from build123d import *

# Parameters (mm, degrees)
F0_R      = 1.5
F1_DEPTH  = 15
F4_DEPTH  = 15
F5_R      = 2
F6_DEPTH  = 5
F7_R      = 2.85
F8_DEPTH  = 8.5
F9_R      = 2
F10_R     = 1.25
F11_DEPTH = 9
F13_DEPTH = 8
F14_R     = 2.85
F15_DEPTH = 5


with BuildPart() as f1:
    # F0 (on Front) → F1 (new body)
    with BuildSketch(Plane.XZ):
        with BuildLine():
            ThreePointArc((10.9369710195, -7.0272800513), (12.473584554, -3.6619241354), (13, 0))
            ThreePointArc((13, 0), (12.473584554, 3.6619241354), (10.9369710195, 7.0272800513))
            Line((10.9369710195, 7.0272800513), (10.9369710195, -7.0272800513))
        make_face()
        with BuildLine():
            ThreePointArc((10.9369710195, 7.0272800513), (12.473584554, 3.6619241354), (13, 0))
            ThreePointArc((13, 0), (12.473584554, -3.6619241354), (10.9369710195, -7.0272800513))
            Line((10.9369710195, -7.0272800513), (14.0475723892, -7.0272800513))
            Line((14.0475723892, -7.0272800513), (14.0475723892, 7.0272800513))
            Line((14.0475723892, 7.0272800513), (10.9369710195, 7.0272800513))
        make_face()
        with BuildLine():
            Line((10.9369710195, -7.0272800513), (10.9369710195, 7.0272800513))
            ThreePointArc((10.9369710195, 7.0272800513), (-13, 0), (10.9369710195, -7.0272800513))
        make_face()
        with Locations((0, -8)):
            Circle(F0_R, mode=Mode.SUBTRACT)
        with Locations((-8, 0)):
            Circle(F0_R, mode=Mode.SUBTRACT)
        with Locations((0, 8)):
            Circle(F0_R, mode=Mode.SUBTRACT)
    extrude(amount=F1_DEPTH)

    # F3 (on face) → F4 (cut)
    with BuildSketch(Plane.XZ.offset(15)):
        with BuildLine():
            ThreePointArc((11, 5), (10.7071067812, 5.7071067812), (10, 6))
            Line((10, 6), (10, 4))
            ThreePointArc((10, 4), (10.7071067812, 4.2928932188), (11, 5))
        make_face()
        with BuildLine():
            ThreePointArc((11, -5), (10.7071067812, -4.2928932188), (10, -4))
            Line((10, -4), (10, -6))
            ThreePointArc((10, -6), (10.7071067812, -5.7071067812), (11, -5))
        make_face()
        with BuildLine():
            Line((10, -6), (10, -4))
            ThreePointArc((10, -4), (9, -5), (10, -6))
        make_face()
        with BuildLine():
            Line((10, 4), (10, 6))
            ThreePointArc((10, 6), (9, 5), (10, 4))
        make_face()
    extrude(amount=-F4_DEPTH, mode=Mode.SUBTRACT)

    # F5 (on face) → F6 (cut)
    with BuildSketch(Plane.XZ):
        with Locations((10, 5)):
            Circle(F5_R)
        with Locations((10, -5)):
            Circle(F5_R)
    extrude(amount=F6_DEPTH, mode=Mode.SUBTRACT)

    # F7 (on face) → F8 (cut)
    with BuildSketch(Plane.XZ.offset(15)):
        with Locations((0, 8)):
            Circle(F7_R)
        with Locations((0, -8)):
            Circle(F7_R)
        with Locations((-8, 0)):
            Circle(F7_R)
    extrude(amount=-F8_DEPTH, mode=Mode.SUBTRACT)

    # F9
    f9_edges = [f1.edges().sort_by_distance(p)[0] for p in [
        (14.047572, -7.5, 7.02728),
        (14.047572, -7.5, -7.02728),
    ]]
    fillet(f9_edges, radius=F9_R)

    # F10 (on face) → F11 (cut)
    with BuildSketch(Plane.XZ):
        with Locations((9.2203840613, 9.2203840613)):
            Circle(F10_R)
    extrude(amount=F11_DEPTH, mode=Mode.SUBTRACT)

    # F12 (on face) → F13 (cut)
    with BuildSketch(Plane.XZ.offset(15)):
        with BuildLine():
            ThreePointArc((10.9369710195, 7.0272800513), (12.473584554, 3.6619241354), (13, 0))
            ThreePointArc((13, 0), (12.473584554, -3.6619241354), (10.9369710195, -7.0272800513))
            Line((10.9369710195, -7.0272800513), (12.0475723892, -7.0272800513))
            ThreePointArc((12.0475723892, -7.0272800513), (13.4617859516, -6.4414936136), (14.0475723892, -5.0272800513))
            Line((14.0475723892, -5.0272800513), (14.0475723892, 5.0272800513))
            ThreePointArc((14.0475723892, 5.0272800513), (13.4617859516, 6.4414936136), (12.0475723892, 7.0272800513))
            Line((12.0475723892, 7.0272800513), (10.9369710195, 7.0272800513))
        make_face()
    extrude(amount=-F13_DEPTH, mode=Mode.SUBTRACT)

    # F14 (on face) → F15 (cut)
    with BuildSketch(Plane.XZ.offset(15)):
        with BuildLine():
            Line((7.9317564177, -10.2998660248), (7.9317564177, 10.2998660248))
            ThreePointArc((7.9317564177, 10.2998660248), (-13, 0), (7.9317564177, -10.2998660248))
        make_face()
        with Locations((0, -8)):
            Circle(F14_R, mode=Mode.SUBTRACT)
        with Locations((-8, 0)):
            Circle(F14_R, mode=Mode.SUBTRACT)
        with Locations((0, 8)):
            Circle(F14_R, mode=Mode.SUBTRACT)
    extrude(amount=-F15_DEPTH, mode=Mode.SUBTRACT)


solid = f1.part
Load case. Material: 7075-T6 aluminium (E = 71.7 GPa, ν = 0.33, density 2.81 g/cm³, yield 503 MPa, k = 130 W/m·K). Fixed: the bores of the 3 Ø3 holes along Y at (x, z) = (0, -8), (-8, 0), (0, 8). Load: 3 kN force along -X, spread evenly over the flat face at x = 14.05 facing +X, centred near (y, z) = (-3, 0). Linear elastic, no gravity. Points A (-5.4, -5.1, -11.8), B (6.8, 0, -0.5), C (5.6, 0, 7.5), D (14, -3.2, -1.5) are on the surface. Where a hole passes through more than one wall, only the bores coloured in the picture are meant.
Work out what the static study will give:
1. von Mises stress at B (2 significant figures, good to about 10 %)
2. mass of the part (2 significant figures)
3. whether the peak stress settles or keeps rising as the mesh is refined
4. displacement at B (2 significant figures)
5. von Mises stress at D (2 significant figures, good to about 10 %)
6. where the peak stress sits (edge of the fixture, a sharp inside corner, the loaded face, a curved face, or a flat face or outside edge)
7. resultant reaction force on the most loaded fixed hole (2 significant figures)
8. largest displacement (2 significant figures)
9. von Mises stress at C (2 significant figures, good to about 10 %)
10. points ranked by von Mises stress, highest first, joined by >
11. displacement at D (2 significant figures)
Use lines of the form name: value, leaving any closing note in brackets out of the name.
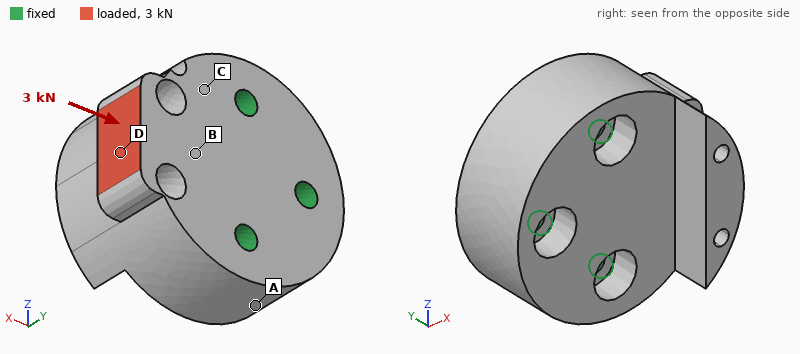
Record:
von Mises stress at B: 49 MPa
mass of the part: 15 g
whether the peak stress settles or keeps rising as the mesh is refined: keeps rising
displacement at B: 5.1 µm
von Mises stress at D: 34 MPa
where the peak stress sits: a sharp inside corner
resultant reaction force on the most loaded fixed hole: 1.3 kN
largest displacement: 12 µm
von Mises stress at C: 19 MPa
points ranked by von Mises stress, highest first, joined by >: B > D > C > A
displacement at D: 9.2 µm
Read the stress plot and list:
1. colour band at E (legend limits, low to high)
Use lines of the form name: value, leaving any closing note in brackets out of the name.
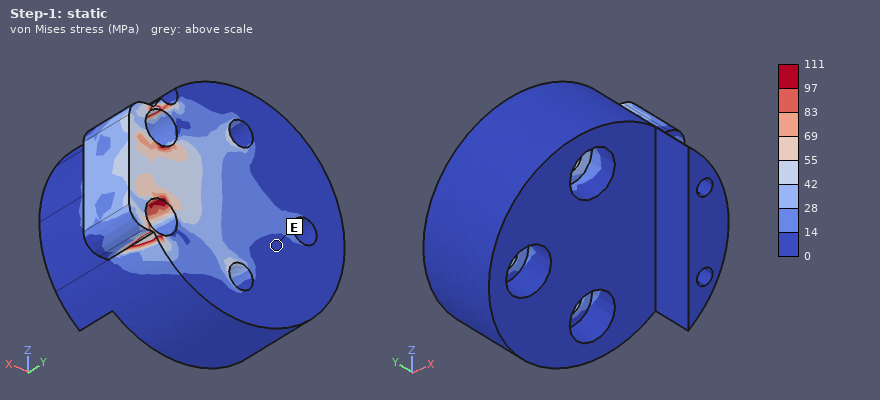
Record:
colour band at E: 0 to 14 MPa
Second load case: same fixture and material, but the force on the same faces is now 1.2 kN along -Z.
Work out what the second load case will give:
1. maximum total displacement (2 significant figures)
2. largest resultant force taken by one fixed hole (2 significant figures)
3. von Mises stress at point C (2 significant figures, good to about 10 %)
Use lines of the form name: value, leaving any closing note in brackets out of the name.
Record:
maximum total displacement: 10 µm
largest resultant force taken by one fixed hole: 1.1 kN
von Mises stress at point C: 12 MPa
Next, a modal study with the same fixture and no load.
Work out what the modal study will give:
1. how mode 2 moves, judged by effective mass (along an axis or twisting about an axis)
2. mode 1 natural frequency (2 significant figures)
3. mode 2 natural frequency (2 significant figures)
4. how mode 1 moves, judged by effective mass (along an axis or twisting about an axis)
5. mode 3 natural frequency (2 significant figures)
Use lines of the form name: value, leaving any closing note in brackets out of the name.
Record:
how mode 2 moves, judged by effective mass: along Z
mode 1 natural frequency: 23 kHz
mode 2 natural frequency: 42 kHz
how mode 1 moves, judged by effective mass: along Y
mode 3 natural frequency: 48 kHz
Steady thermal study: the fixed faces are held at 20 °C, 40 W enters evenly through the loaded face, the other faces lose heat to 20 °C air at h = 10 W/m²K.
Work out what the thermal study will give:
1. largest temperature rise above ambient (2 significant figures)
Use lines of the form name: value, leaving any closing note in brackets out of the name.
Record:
largest temperature rise above ambient: 41 K
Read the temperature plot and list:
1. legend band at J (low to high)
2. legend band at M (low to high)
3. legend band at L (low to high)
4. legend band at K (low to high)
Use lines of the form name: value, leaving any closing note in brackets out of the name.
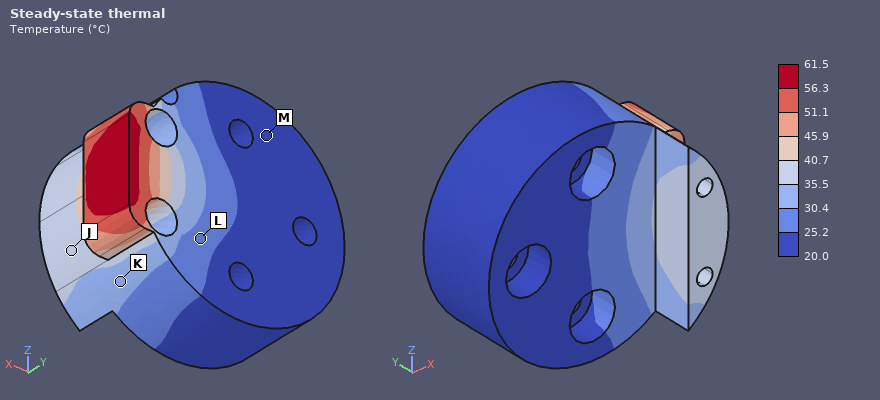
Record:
legend band at J: 35.5 to 40.7 °C
legend band at M: 20.0 to 25.2 °C
legend band at L: 25.2 to 30.4 °C
legend band at K: 30.4 to 35.5 °C
